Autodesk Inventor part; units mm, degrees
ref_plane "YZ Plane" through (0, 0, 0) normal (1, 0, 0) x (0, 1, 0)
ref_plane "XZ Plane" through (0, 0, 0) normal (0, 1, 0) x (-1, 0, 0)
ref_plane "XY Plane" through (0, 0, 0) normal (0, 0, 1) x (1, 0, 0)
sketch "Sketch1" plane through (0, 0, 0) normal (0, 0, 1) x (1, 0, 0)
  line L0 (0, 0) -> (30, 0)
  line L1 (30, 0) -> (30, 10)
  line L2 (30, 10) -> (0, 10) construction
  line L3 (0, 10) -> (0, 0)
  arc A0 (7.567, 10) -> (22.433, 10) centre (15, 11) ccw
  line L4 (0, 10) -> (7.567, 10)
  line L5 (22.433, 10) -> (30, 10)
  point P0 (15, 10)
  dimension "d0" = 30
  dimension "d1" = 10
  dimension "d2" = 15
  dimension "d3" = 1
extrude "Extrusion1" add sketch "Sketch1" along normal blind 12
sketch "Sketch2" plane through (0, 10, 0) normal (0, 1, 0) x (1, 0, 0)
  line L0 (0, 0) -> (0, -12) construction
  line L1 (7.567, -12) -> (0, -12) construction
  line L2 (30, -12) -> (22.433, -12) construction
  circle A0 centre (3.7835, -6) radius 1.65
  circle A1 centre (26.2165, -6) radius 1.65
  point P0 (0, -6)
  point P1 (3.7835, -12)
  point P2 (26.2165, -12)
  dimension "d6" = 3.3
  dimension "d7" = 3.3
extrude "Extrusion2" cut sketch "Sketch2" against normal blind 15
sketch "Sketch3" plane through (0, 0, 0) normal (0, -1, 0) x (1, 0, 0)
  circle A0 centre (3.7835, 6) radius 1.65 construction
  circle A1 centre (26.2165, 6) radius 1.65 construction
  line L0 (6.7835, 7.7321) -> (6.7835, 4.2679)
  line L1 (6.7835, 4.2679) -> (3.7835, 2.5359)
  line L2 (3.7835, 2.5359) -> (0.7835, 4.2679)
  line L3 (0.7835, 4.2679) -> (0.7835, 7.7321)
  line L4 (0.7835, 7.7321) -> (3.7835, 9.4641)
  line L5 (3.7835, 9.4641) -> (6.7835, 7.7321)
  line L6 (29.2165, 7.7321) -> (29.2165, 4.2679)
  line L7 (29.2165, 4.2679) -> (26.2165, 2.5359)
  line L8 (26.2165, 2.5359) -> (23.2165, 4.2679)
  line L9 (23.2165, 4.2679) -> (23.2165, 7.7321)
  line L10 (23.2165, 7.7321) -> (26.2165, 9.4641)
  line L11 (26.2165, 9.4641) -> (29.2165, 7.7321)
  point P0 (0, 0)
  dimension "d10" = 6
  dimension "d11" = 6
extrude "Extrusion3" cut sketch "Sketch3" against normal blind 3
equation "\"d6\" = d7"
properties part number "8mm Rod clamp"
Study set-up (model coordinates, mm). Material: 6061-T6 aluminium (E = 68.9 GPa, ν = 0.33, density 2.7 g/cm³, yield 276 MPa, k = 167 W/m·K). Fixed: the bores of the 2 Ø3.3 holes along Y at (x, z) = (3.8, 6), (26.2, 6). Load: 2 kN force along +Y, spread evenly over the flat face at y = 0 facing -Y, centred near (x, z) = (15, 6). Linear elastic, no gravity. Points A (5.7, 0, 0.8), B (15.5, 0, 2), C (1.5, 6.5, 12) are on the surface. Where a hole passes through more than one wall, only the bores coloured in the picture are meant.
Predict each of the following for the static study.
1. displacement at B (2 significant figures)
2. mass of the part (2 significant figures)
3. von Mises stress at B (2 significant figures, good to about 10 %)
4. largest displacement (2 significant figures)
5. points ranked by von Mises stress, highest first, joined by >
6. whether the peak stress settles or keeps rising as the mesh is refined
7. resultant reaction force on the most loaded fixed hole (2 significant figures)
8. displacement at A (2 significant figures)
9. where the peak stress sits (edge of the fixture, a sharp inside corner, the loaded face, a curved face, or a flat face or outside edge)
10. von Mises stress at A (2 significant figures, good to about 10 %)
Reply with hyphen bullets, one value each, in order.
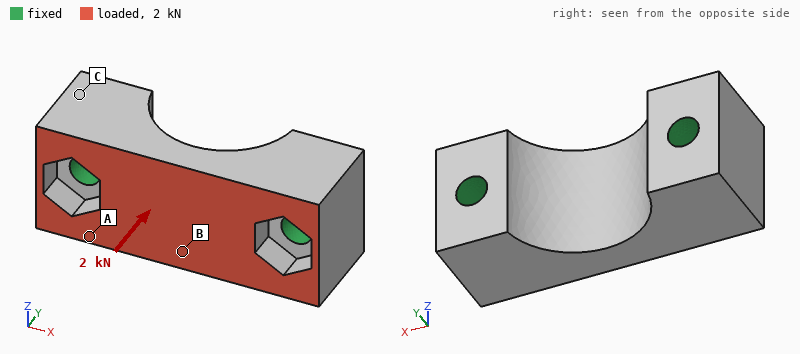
- 5.6 µm
- 6.5 g
- 25 MPa
- 6.0 µm
- B > A > C
- keeps rising
- 1.1 kN
- 2.5 µm
- edge of the fixture
- 10 MPa
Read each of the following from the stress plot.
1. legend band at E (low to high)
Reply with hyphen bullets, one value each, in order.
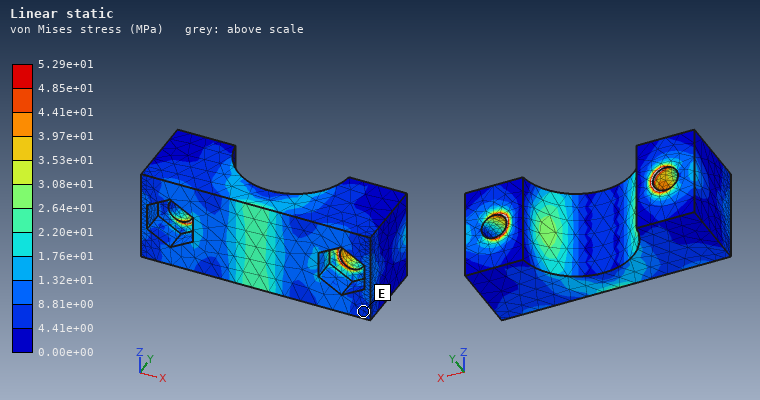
- 4.41e+00 to 8.81e+00 MPa
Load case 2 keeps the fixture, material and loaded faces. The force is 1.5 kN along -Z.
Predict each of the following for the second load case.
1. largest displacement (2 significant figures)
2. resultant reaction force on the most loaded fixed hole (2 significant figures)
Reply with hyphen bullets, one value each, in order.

- 13 µm
- 750 N
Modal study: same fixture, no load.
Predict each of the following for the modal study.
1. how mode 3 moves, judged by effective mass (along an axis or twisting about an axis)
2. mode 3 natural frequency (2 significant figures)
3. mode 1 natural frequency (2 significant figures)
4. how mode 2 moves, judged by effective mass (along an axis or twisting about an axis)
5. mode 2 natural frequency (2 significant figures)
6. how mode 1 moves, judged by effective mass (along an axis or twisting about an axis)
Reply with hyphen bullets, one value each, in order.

- twisting about X
- 67 kHz
- 41 kHz
- along Y
- 56 kHz
- along Z
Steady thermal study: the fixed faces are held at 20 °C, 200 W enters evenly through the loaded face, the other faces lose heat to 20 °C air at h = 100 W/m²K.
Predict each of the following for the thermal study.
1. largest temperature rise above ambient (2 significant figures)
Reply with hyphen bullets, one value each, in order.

- 62 K
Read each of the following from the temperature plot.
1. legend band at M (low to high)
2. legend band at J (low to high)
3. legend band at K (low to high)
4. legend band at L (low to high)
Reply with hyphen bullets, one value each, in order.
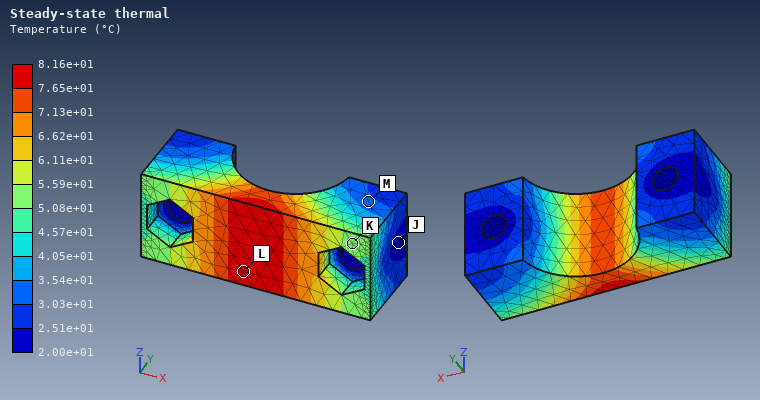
- 3.03e+01 to 3.54e+01 °C
- 2.00e+01 to 2.51e+01 °C
- 5.08e+01 to 5.59e+01 °C
- 7.65e+01 to 8.16e+01 °C
